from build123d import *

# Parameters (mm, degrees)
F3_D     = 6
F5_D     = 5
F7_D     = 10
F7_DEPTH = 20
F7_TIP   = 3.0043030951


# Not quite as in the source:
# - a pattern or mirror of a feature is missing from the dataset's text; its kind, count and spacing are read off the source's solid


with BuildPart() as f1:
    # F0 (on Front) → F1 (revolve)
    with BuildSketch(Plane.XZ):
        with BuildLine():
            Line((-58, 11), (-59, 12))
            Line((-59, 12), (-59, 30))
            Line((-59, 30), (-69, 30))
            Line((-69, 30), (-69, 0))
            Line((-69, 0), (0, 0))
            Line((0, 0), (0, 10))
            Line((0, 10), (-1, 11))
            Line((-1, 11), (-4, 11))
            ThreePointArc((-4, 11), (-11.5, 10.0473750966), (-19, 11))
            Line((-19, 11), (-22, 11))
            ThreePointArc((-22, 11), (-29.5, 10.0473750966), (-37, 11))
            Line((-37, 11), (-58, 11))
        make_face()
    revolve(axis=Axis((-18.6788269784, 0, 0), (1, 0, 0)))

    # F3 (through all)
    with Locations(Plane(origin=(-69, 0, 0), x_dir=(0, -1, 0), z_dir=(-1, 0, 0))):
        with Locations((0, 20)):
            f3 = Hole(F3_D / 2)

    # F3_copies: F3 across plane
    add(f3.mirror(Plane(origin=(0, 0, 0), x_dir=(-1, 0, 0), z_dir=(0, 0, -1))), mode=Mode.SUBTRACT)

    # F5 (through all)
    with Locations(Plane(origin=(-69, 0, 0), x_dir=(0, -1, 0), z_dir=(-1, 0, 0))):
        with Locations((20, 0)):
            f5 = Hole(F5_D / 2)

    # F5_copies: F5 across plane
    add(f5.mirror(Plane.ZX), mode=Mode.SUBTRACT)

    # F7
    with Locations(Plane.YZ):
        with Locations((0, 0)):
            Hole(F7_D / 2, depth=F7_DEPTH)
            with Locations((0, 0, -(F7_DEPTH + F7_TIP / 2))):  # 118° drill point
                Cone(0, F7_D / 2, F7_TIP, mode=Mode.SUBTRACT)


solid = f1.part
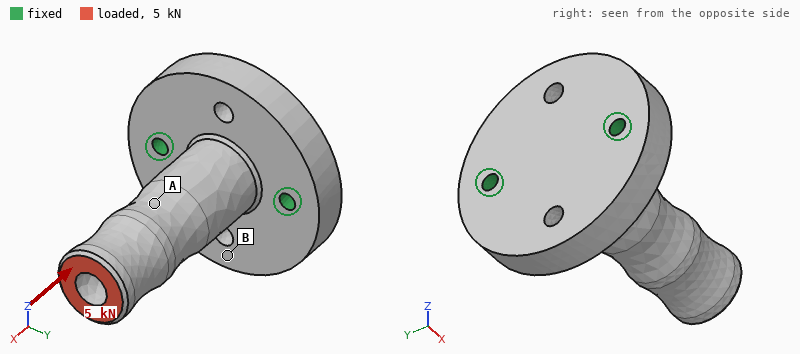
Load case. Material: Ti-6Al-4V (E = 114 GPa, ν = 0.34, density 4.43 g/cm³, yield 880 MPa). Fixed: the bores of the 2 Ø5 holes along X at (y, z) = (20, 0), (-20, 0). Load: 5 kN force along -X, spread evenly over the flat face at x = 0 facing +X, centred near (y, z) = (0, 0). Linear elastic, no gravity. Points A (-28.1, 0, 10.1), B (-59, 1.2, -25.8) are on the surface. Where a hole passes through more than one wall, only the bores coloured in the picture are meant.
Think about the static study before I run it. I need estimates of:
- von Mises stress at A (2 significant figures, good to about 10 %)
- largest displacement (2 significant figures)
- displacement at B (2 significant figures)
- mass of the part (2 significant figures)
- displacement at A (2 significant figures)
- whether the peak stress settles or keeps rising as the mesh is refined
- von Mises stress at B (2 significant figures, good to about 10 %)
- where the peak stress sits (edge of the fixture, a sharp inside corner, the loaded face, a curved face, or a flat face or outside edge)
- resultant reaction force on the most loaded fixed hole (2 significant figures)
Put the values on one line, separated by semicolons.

18 MPa; 15 µm; 7.3 µm; 210 g; 9.9 µm; keeps rising; 8.9 MPa; edge of the fixture; 2.6 kN
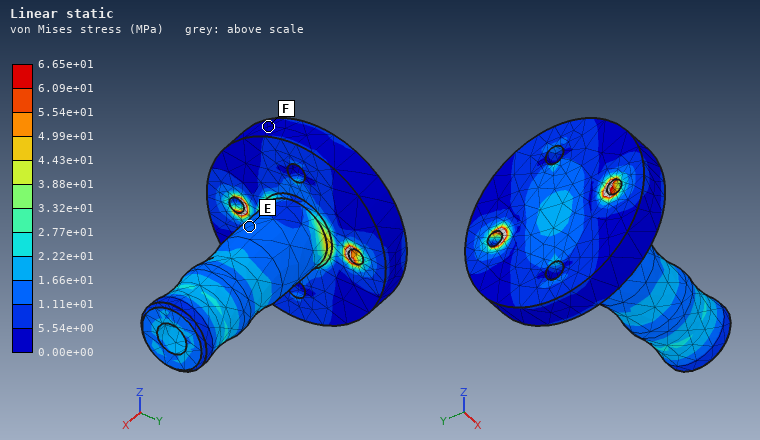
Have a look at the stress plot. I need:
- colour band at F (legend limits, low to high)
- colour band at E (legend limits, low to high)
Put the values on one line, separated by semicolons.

0.00e+00 to 5.54e+00 MPa; 1.11e+01 to 1.66e+01 MPa
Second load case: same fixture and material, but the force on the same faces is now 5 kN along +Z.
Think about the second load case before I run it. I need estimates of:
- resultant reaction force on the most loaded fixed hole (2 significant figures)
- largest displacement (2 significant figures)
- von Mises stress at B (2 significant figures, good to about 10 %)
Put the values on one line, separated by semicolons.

2.5 kN; 0.70 mm; 65 MPa
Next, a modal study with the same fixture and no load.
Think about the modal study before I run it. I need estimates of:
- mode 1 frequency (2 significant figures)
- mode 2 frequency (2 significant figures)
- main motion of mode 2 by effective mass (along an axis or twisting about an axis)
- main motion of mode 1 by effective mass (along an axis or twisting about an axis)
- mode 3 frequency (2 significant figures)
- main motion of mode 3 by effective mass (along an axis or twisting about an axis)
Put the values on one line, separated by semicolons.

2700 Hz; 3900 Hz; along Y; along Z; 9800 Hz; along X
